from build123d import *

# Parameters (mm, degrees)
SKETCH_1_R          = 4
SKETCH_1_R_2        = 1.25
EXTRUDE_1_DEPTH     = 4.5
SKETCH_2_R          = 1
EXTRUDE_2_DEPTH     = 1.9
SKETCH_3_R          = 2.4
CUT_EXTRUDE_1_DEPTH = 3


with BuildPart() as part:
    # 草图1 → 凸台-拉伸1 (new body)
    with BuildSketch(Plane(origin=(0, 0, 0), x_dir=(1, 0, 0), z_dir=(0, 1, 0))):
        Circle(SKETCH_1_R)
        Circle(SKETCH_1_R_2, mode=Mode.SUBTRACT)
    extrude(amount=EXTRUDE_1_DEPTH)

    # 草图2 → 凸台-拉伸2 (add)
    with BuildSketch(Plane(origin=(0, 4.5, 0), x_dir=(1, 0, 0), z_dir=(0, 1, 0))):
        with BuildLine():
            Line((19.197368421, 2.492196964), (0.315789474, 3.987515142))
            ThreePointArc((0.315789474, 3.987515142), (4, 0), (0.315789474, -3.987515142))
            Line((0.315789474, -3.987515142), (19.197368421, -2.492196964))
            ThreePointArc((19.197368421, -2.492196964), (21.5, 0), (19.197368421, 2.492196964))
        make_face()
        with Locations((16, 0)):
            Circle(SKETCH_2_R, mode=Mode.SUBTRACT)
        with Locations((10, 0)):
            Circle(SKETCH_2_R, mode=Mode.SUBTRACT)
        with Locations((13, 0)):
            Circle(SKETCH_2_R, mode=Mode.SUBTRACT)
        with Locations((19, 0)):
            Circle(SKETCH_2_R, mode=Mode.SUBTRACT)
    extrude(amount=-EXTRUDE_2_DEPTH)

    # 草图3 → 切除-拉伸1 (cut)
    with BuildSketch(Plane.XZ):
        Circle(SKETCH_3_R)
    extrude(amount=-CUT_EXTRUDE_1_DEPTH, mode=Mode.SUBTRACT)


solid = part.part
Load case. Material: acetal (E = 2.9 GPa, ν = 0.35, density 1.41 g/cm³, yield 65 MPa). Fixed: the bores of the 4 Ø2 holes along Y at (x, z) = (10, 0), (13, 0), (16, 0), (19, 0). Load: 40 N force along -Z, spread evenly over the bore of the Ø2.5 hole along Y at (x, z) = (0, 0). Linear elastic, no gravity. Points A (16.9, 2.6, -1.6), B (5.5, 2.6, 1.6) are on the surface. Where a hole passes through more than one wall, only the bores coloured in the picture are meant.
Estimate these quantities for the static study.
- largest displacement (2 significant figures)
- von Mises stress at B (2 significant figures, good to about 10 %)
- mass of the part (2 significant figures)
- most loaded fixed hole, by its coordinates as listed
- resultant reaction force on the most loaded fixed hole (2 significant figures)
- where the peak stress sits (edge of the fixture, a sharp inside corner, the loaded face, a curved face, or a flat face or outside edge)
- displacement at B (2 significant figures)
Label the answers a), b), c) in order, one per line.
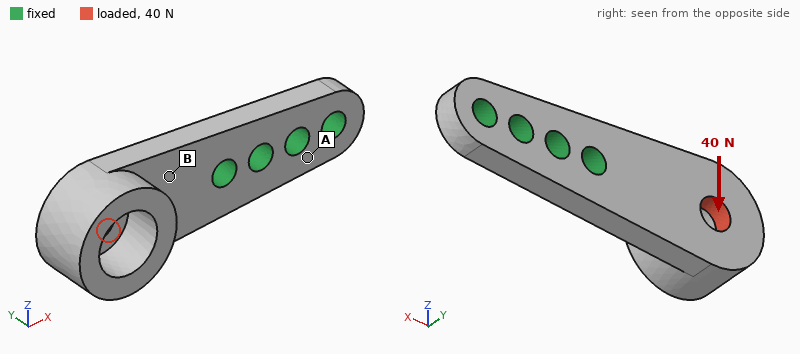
a) 0.27 mm
b) 8.0 MPa
c) 0.49 g
d) (10, 0)
e) 85 N
f) edge of the fixture
g) 0.067 mm
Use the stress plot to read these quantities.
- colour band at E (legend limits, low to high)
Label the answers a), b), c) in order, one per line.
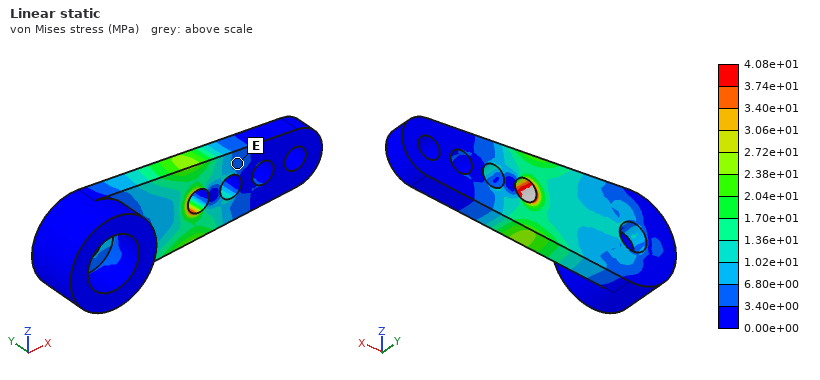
a) 3.40e+00 to 6.80e+00 MPa
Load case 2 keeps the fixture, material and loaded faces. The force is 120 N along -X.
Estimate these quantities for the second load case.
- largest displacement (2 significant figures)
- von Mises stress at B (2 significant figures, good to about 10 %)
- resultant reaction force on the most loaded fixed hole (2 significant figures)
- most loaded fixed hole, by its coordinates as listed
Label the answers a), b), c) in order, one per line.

a) 0.17 mm
b) 4.2 MPa
c) 97 N
d) (10, 0)
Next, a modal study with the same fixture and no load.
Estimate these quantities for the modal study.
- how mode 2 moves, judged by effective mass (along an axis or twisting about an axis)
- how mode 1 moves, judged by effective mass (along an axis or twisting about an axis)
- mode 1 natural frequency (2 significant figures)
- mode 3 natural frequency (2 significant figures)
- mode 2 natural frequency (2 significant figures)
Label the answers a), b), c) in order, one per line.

a) along Z
b) along Y
c) 1900 Hz
d) 6000 Hz
e) 4200 Hz
